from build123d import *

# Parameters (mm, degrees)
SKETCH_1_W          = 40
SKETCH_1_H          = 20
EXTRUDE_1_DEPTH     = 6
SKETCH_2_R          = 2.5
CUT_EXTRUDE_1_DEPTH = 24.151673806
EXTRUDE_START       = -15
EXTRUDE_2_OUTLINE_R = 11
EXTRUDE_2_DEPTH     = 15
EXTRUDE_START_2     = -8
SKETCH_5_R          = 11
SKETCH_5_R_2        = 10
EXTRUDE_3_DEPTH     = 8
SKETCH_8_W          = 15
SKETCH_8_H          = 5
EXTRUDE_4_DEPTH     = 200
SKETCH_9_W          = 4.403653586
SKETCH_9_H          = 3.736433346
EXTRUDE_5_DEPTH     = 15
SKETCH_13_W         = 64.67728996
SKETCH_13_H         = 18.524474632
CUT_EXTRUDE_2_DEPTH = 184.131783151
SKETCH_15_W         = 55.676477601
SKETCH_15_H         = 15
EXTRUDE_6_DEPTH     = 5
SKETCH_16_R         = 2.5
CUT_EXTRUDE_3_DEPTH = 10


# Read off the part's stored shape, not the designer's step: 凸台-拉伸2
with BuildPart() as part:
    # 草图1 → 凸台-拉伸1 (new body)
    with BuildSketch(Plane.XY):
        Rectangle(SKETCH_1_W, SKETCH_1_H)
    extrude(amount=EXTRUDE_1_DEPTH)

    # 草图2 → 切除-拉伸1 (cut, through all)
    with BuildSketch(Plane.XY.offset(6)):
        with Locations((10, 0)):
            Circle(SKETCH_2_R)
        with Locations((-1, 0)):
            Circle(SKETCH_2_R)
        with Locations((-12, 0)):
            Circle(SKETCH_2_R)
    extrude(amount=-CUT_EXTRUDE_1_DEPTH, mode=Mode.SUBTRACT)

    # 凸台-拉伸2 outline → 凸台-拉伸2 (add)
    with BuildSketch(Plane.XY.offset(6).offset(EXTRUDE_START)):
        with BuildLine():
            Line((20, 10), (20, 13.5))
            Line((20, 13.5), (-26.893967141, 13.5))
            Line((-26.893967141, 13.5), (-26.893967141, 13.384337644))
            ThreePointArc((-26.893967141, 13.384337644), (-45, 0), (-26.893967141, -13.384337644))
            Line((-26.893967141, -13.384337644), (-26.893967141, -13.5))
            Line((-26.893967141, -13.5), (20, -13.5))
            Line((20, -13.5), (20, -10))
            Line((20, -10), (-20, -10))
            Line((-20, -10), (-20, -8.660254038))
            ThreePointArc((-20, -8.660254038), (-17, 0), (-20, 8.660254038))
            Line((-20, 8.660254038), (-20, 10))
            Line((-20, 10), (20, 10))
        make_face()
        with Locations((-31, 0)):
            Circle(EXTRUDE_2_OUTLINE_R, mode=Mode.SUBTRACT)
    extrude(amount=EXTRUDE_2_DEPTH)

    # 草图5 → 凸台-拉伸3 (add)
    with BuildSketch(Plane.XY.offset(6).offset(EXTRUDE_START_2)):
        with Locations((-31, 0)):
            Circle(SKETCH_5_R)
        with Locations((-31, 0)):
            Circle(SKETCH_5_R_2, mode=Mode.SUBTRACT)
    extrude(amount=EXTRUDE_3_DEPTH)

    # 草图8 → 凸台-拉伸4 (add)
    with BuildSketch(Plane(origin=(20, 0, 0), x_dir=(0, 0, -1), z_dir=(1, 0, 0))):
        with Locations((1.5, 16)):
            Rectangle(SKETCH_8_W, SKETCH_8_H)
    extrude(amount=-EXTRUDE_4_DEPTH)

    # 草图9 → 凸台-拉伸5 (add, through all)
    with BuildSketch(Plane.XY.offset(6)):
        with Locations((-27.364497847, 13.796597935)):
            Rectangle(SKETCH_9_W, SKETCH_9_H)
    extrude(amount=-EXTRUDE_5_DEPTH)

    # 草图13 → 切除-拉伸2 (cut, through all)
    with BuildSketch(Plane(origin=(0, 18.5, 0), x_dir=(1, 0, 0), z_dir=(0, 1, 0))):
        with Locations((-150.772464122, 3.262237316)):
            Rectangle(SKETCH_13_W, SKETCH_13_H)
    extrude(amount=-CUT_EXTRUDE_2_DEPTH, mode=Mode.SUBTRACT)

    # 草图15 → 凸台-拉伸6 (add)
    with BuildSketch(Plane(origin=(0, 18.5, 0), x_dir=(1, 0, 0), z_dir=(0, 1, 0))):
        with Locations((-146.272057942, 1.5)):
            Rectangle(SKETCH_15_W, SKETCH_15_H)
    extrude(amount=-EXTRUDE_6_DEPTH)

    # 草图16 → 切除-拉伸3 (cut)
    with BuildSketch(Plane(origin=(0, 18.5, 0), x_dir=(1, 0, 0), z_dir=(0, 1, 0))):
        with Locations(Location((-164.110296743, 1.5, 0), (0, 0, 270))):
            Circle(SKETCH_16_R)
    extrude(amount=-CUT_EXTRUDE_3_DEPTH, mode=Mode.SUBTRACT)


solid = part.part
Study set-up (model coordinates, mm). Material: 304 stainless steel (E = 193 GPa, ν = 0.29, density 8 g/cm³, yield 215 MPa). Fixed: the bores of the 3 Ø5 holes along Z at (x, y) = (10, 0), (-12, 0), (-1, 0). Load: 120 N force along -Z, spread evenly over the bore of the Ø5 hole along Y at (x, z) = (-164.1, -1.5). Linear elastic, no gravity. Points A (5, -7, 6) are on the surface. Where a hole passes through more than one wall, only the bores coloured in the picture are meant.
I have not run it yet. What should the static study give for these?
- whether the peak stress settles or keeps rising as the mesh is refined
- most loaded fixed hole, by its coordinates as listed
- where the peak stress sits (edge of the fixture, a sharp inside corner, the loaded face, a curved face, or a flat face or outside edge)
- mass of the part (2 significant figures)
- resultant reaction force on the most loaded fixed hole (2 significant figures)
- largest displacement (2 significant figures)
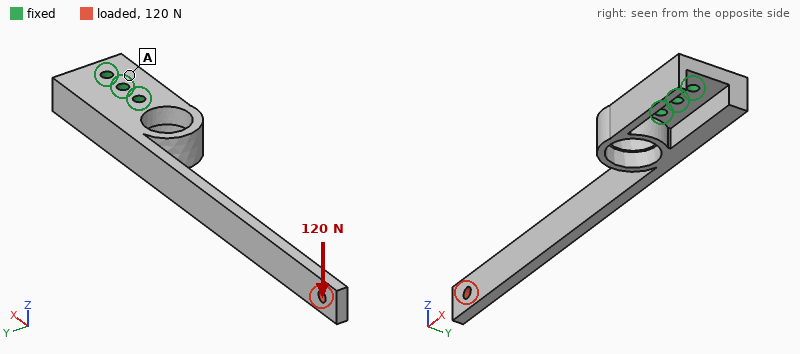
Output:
keeps rising
(-12, 0)
edge of the fixture
220 g
800 N
0.53 mm
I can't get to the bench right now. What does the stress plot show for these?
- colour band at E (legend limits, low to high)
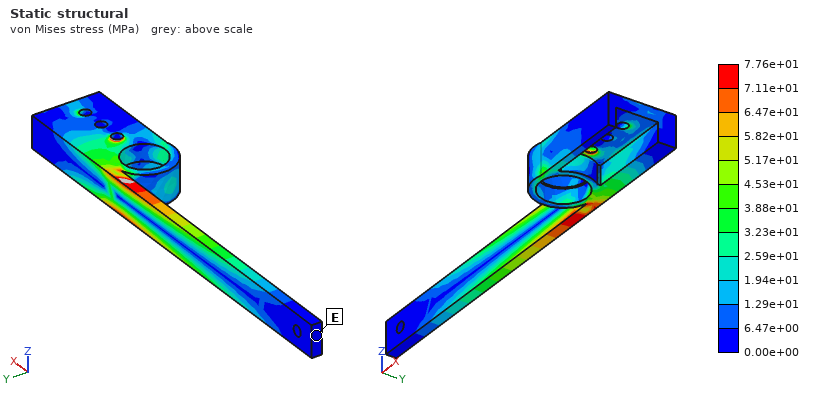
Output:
0.00e+00 to 6.47e+00 MPa
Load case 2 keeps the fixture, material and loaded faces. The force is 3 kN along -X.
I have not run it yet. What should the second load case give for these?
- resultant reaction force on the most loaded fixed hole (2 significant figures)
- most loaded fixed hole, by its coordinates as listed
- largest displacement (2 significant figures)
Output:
2.2 kN
(-12, 0)
0.12 mm
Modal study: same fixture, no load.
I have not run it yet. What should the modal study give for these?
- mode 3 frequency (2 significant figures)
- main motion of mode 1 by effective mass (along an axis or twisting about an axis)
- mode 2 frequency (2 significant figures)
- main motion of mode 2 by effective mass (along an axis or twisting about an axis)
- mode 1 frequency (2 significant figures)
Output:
1200 Hz
along Y
480 Hz
along Z
200 Hz
